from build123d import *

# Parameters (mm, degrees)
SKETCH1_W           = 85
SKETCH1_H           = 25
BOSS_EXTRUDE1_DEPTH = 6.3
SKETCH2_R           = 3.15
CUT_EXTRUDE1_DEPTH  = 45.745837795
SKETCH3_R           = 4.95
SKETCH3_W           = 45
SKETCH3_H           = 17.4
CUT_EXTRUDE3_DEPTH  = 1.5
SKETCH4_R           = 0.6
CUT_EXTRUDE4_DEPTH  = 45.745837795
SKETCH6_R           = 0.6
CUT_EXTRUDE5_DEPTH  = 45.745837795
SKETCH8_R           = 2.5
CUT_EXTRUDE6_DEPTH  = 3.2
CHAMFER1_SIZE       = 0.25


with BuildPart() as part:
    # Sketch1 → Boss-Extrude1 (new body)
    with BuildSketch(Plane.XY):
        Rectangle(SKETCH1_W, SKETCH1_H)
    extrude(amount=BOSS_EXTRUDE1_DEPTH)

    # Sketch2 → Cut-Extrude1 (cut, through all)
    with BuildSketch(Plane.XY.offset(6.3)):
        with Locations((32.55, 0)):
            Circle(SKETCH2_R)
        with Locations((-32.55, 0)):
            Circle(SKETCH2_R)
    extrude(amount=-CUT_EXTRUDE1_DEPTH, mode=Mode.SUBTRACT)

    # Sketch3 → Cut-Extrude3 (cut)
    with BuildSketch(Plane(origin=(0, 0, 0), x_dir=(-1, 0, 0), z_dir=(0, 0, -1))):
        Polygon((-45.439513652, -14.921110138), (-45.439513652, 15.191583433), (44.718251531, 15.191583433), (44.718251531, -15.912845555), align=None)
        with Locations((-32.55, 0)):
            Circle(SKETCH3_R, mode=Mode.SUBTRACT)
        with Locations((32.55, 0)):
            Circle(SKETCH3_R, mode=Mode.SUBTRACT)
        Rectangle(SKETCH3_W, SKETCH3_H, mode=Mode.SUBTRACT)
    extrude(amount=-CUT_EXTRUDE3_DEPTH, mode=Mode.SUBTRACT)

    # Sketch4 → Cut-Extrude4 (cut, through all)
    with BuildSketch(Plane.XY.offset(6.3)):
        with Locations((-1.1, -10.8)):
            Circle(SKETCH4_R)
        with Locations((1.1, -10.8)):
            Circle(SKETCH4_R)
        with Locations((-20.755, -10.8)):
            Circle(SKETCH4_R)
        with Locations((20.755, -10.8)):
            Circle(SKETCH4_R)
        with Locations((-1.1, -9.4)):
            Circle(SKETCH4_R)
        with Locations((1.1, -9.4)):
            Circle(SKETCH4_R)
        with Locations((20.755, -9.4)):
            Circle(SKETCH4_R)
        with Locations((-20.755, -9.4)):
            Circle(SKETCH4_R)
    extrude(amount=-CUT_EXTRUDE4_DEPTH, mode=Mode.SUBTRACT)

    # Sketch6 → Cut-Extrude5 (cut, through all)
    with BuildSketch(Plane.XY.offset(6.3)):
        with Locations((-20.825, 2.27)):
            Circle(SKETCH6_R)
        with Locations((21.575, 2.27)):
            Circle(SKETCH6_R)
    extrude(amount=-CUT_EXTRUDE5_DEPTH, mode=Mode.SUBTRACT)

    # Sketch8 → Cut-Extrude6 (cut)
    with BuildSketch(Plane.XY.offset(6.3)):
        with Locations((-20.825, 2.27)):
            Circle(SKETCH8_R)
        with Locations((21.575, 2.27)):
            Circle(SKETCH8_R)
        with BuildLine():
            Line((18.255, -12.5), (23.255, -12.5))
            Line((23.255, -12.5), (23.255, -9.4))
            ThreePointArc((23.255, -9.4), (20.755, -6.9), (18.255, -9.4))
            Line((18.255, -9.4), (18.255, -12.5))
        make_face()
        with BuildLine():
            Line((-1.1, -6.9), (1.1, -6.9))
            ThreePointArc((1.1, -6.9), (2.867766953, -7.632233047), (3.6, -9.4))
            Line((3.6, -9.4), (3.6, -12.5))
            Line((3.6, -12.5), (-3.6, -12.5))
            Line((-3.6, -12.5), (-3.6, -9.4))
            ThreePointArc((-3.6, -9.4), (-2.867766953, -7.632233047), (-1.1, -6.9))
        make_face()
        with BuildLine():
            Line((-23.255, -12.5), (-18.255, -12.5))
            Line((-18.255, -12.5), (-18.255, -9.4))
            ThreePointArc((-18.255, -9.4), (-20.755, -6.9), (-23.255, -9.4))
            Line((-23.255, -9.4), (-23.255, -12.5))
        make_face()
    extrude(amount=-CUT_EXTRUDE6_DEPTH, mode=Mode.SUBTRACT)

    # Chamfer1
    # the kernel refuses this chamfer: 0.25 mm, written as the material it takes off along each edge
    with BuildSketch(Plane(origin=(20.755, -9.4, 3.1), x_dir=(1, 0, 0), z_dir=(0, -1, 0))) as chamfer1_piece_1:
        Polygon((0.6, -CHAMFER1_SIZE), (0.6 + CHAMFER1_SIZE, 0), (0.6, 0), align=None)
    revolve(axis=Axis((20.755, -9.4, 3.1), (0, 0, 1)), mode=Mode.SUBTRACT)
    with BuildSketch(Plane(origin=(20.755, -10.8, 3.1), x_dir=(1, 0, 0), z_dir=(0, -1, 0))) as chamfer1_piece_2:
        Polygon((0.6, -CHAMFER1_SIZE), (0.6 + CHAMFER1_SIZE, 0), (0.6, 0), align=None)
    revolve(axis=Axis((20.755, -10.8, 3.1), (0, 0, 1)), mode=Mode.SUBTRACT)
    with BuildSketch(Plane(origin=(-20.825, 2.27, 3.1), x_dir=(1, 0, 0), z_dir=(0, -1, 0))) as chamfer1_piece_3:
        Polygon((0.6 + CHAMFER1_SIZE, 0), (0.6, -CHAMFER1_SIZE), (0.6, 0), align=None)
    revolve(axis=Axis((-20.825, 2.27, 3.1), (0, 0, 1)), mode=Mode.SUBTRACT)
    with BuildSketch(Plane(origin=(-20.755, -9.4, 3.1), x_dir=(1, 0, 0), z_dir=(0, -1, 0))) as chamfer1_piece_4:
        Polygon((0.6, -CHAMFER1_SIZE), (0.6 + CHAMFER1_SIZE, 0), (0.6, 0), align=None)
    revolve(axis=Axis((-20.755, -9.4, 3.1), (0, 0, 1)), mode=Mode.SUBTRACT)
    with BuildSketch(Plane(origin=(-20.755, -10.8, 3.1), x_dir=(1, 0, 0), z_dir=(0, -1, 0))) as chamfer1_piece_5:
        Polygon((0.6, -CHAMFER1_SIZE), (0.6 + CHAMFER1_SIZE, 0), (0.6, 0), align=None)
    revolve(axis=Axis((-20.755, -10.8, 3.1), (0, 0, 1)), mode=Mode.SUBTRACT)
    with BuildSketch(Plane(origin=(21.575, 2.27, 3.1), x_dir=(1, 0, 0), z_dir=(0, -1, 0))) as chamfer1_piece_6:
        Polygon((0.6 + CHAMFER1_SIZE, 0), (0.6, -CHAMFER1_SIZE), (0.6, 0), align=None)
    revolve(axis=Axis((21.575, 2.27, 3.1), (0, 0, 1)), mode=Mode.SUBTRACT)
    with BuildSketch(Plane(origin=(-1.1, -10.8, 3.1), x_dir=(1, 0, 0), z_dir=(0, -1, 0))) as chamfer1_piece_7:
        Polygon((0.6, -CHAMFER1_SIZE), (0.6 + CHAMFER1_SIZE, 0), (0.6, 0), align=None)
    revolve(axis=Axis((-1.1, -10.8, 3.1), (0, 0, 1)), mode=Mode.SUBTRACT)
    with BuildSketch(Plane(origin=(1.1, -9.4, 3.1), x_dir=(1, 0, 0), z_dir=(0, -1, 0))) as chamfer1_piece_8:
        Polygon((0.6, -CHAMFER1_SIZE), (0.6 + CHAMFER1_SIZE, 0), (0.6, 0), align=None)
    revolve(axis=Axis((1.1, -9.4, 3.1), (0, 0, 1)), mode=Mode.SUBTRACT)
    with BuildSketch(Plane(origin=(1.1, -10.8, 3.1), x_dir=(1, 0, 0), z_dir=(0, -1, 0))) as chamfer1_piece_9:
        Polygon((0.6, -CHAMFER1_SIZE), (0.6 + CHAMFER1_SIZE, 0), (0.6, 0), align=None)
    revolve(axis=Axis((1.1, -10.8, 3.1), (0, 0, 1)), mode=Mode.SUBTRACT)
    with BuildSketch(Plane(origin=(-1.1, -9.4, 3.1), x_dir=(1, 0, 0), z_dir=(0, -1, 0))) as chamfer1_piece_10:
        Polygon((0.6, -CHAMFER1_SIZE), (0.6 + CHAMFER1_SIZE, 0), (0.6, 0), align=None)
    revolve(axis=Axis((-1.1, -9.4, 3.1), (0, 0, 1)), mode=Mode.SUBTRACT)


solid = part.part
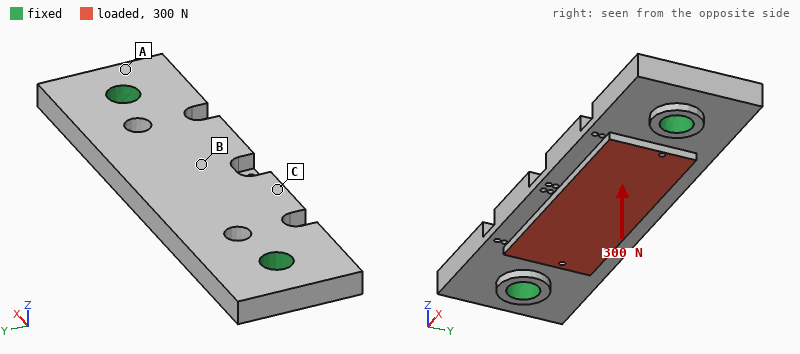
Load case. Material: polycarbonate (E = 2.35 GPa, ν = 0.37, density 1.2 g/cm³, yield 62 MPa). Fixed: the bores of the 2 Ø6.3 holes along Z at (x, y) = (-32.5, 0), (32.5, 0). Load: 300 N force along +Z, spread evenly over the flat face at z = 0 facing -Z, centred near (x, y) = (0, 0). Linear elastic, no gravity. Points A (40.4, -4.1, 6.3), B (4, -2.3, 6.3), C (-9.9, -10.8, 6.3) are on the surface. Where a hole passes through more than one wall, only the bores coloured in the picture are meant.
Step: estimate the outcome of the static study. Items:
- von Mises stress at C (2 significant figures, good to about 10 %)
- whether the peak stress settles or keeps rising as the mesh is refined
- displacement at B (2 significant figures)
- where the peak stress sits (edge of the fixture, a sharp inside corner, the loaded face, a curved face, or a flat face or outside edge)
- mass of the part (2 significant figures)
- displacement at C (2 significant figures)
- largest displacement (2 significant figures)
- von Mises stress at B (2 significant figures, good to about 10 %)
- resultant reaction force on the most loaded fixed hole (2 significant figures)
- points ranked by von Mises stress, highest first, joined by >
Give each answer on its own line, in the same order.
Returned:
4.4 MPa
keeps rising
0.37 mm
edge of the fixture
13 g
0.34 mm
0.43 mm
9.1 MPa
170 N
B > C > A
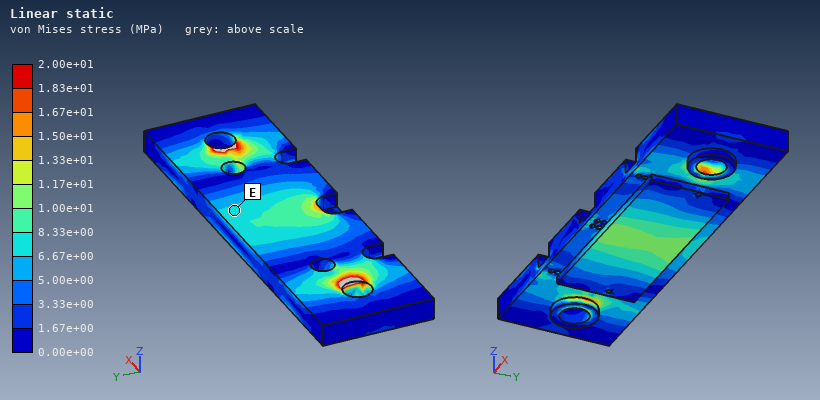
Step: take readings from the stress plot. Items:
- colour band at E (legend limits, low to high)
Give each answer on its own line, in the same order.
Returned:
6.67e+00 to 8.33e+00 MPa
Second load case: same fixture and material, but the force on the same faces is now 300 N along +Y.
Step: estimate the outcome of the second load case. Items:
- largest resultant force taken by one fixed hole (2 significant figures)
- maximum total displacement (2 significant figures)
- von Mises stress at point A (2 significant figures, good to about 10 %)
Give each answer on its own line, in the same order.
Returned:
150 N
0.18 mm
1.3 MPa
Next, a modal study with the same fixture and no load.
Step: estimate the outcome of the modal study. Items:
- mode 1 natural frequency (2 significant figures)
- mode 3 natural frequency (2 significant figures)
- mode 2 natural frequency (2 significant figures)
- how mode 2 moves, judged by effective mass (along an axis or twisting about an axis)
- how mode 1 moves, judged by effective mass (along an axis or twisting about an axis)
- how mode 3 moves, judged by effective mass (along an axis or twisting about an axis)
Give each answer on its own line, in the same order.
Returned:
1800 Hz
3600 Hz
2700 Hz
twisting about X
along Z
along Y
